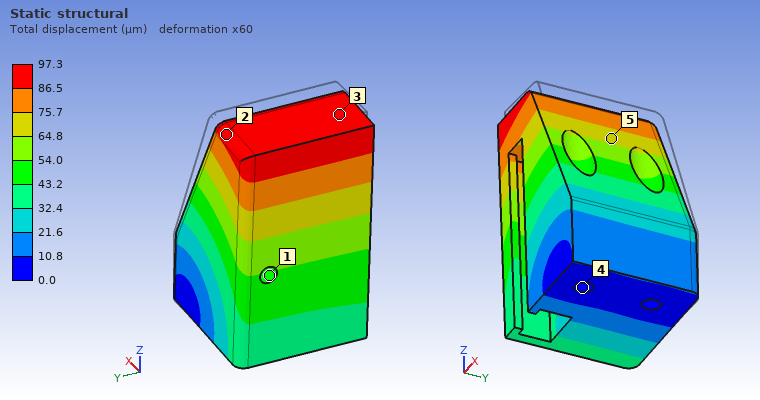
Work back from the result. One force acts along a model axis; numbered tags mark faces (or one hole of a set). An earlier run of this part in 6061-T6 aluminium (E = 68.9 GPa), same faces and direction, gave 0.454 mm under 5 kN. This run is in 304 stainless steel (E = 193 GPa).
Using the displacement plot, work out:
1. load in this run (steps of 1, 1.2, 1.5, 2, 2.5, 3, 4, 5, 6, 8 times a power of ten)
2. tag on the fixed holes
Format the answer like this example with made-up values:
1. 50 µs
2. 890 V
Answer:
1. 3 kN
2. 4
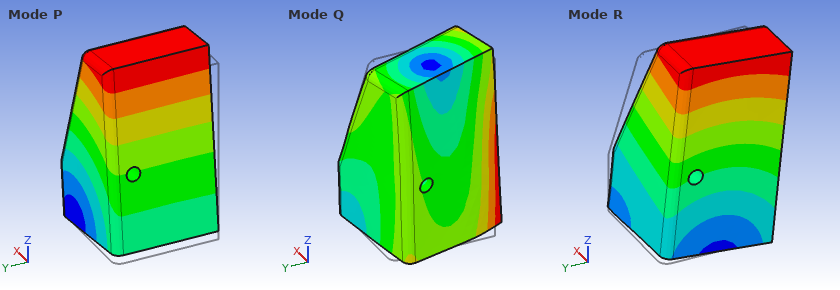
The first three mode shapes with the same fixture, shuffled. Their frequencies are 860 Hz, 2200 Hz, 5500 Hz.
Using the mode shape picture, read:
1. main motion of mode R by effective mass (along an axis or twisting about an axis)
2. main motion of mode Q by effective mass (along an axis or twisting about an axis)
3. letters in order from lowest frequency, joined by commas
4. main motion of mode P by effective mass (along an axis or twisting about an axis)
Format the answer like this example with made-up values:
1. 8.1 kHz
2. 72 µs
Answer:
1. along Y
2. twisting about Z
3. P, R, Q
4. along X
